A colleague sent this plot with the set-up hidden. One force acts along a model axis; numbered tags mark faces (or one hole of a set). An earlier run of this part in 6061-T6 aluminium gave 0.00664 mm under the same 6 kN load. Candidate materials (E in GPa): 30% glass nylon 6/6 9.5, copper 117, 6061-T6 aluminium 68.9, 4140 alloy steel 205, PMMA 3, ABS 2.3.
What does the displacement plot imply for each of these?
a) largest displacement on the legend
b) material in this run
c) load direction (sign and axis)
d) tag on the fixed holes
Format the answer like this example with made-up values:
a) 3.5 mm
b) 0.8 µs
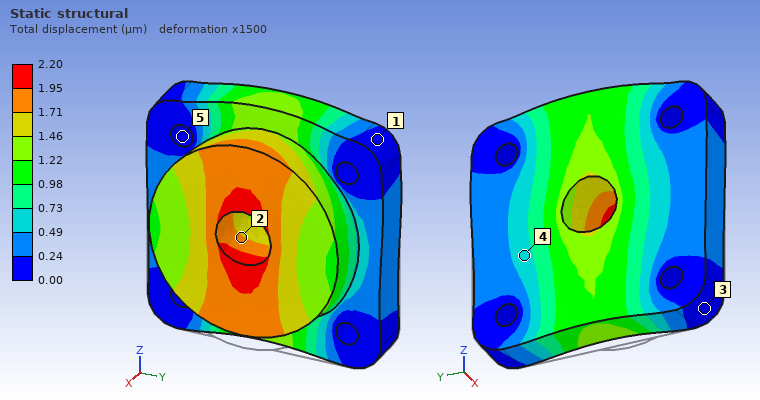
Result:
a) 2.20 µm
b) 4140 alloy steel
c) +Z
d) 5
